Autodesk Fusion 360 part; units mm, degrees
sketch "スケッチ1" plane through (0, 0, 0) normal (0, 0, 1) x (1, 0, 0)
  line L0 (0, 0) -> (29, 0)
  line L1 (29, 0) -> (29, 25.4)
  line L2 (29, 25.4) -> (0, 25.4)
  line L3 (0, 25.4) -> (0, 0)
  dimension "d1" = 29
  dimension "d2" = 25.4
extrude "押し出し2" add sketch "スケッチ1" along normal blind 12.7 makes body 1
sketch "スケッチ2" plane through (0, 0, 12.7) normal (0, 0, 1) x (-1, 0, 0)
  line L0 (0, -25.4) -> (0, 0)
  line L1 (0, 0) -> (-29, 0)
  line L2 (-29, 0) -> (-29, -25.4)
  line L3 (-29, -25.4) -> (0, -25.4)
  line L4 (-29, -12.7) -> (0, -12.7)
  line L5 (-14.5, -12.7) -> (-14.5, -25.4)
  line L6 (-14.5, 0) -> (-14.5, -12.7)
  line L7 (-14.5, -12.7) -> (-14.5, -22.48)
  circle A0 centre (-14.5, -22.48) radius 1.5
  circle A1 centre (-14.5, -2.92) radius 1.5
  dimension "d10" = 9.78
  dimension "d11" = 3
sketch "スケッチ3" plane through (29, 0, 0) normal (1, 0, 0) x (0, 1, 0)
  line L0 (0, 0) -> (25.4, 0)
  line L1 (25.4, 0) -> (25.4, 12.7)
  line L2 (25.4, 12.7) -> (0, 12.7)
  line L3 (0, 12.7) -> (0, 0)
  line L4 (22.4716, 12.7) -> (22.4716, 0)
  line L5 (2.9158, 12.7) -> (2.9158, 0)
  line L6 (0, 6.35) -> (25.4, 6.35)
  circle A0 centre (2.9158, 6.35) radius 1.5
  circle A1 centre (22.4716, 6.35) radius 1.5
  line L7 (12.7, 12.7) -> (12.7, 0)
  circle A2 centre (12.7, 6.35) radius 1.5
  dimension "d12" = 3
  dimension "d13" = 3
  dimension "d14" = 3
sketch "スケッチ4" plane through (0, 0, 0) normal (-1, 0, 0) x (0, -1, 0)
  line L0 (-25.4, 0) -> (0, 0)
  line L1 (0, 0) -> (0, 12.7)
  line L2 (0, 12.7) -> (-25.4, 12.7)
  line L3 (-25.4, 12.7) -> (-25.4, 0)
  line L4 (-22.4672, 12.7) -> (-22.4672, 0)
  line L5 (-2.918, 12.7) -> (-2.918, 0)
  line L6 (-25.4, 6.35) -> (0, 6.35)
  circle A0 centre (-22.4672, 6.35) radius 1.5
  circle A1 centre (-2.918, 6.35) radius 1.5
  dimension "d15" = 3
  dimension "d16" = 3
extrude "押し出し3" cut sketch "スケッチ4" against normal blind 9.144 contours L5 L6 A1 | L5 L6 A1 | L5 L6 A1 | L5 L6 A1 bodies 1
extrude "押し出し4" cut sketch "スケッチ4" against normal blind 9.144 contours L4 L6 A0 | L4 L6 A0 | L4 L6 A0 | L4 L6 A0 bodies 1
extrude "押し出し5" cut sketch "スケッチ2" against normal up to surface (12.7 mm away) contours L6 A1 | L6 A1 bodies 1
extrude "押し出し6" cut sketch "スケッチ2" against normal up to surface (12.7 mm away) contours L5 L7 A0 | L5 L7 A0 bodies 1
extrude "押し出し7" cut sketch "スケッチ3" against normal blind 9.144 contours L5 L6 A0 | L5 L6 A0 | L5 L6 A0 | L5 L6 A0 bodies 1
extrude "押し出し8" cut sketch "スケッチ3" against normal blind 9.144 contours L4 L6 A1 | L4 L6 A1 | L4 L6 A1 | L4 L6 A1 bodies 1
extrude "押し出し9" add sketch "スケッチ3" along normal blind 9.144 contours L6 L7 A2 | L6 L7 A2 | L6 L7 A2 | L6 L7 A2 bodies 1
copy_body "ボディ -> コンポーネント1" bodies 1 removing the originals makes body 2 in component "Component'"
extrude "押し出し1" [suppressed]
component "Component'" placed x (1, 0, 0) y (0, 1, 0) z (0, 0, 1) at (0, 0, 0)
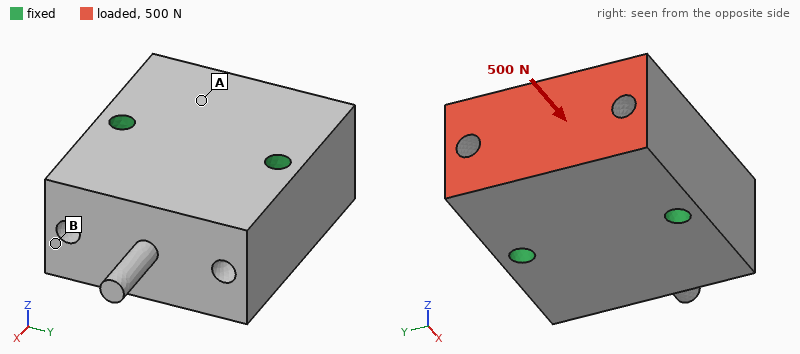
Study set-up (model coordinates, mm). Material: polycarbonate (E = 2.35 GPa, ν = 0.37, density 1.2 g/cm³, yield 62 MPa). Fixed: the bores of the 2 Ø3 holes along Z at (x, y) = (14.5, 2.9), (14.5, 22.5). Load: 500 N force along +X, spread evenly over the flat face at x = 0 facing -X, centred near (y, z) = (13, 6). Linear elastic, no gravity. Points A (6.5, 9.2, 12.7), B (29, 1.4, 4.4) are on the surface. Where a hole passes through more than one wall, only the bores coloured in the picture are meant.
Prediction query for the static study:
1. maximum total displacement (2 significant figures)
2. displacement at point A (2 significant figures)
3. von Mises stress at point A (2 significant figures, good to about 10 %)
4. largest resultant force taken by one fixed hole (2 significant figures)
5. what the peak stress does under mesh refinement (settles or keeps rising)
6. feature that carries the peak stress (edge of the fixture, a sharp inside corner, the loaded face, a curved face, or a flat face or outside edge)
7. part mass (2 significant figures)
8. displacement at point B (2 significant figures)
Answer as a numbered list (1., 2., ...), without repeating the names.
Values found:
1. 12 µm
2. 8.2 µm
3. 1.3 MPa
4. 250 N
5. keeps rising
6. edge of the fixture
7. 11 g
8. 1.9 µm
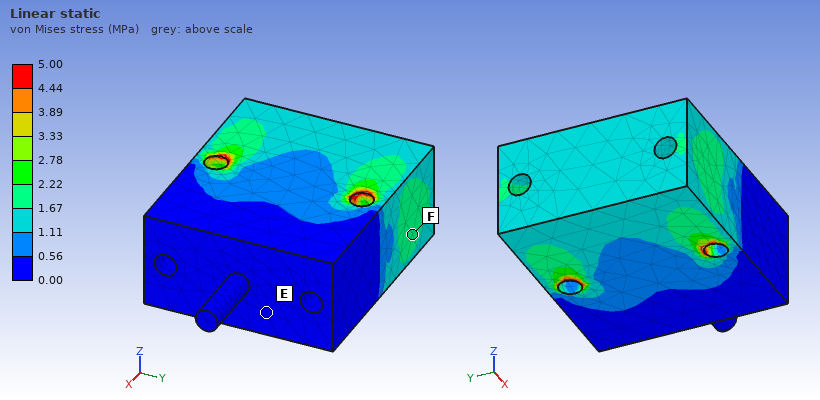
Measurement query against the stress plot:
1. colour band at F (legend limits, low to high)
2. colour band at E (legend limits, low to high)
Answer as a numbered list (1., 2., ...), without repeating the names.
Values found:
1. 1.67 to 2.22 MPa
2. 0.00 to 0.56 MPa
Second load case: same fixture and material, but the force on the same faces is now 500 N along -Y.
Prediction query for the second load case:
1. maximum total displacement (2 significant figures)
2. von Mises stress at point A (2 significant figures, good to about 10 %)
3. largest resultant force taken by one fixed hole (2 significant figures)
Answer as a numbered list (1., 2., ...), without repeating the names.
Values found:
1. 58 µm
2. 4.1 MPa
3. 420 N
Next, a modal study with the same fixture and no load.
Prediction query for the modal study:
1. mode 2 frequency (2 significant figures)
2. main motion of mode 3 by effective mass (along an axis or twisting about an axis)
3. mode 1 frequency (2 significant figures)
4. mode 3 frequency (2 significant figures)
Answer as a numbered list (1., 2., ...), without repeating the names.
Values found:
1. 5900 Hz
2. twisting about Y
3. 5700 Hz
4. 7500 Hz
